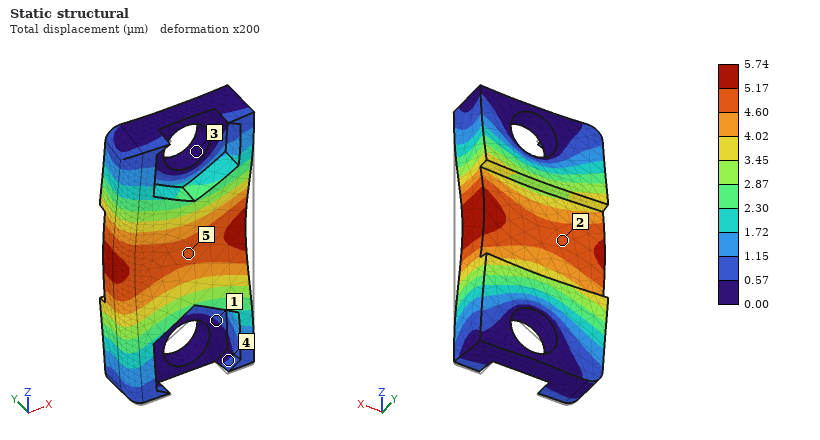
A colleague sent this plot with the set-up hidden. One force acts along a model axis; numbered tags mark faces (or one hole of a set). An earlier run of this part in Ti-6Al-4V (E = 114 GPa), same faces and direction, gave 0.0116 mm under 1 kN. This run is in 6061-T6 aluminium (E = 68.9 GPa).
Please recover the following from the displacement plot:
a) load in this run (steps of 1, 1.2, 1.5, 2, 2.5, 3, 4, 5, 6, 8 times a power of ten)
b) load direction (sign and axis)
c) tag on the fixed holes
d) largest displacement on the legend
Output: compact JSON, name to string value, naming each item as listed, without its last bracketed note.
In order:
{"load in this run": "300 N", "load direction": "+Y", "tag on the fixed holes": "3", "largest displacement on the legend": "5.74 µm"}
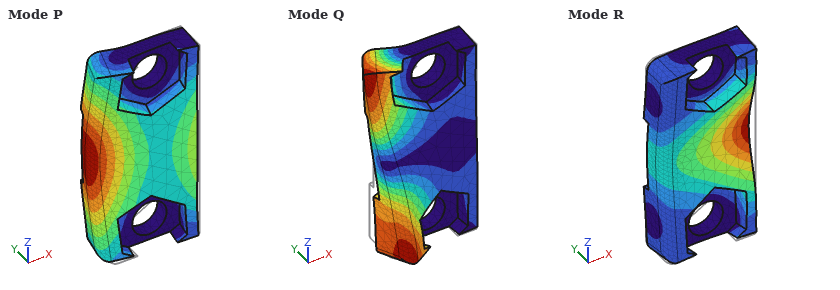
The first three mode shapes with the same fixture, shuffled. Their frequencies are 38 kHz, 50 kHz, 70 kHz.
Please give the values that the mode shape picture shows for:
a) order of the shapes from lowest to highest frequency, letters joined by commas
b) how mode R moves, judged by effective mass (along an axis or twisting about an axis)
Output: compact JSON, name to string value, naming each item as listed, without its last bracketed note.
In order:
{"order of the shapes from lowest to highest frequency, letters joined by commas": "P, R, Q", "how mode R moves, judged by effective mass": "along Y"}
